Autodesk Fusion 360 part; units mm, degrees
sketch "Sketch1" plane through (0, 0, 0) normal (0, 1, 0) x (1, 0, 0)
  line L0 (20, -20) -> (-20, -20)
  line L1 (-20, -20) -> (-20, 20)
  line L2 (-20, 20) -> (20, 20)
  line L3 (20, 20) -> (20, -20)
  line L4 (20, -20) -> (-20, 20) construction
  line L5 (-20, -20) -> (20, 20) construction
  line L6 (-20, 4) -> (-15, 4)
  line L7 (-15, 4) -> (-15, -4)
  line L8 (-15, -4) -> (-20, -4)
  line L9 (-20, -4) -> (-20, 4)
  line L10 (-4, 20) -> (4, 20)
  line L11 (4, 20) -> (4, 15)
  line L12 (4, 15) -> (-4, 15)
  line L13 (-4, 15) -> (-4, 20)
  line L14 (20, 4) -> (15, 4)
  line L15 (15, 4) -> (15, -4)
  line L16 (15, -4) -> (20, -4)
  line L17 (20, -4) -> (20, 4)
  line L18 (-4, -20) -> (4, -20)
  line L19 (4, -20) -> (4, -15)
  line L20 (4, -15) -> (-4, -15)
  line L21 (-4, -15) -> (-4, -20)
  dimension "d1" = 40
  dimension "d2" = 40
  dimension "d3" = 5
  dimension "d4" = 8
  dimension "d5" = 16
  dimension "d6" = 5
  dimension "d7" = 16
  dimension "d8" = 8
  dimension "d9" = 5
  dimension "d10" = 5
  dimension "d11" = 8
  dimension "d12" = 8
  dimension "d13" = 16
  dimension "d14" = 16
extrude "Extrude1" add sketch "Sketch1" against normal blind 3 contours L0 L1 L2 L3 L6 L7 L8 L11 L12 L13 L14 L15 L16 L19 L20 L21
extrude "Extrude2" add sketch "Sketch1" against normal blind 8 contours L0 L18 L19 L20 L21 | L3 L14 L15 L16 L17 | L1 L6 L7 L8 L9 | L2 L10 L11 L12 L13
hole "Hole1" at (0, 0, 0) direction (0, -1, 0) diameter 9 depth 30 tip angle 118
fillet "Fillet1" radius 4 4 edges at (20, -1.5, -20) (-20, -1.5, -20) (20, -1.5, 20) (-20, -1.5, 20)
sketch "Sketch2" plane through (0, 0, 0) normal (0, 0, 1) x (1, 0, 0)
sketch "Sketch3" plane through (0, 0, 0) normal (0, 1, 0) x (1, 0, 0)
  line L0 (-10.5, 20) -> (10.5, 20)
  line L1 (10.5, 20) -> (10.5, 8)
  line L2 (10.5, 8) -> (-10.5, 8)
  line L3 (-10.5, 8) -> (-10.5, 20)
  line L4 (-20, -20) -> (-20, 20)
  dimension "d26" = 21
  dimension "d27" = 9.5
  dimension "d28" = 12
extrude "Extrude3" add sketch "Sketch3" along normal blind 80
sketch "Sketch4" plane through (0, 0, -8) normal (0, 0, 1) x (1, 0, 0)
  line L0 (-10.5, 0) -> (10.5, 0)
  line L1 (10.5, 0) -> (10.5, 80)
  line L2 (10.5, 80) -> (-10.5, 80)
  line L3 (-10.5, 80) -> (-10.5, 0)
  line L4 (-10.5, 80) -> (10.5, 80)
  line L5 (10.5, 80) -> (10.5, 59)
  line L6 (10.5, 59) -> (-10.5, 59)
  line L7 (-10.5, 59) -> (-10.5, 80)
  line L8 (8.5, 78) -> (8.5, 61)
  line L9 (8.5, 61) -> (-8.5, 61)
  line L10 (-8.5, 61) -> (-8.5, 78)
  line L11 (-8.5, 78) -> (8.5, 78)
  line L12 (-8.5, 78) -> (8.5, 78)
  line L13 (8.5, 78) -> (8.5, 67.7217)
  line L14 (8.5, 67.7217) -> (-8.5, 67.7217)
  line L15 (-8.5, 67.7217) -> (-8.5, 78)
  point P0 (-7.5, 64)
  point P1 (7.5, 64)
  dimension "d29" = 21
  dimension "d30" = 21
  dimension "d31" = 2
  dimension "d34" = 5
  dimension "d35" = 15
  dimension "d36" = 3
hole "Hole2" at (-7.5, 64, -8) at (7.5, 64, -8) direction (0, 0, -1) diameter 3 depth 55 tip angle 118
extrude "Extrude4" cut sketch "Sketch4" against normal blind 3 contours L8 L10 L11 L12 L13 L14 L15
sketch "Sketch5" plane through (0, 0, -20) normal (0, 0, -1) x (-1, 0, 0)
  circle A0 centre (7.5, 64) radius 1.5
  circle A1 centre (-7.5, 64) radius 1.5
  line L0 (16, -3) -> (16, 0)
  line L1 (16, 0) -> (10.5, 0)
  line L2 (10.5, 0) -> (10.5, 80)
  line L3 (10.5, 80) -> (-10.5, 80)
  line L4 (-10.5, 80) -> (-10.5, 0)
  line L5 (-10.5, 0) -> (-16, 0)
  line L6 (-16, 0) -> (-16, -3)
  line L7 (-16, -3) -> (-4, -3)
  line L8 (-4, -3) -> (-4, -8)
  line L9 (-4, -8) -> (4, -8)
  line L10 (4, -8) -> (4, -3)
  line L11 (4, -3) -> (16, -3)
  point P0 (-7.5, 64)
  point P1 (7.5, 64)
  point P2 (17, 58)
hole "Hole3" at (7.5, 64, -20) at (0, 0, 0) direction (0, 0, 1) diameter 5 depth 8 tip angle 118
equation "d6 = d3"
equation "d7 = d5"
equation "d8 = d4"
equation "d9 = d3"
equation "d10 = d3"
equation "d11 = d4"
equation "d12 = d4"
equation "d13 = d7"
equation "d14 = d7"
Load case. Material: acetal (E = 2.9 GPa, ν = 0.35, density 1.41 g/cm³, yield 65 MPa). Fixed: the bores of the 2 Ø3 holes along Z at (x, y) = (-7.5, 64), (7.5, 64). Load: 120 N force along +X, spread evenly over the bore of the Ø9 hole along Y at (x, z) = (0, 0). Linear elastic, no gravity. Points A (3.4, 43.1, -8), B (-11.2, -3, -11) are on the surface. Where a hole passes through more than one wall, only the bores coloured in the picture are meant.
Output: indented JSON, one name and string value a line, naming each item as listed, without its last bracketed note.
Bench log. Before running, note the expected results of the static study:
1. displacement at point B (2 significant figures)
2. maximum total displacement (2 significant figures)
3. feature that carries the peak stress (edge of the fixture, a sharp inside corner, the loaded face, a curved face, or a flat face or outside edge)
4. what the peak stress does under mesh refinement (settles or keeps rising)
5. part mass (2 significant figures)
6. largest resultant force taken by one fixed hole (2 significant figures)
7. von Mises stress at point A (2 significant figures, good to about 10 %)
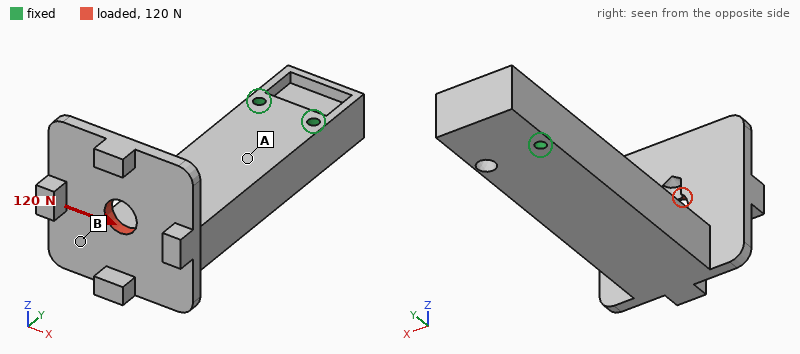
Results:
{
  "displacement at point B": "0.64 mm",
  "maximum total displacement": "1.2 mm",
  "feature that carries the peak stress": "edge of the fixture",
  "what the peak stress does under mesh refinement": "keeps rising",
  "part mass": "35 g",
  "largest resultant force taken by one fixed hole": "460 N",
  "von Mises stress at point A": "5.4 MPa"
}
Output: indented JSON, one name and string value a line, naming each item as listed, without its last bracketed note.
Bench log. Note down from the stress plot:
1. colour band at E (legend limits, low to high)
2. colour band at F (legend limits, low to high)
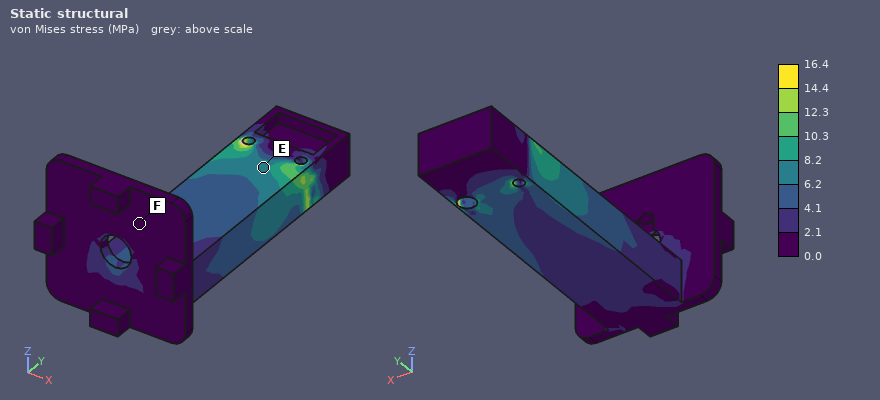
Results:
{
  "colour band at E": "6.2 to 8.2 MPa",
  "colour band at F": "0.0 to 2.1 MPa"
}
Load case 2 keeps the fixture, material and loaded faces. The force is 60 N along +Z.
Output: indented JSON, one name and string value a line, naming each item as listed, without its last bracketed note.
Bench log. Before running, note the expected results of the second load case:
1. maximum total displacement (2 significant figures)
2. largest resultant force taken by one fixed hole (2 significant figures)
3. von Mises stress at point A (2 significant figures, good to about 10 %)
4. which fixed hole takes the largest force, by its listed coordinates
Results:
{
  "maximum total displacement": "1.1 mm",
  "largest resultant force taken by one fixed hole": "64 N",
  "von Mises stress at point A": "5.2 MPa",
  "which fixed hole takes the largest force, by its listed coordinates": "(-7.5, 64)"
}
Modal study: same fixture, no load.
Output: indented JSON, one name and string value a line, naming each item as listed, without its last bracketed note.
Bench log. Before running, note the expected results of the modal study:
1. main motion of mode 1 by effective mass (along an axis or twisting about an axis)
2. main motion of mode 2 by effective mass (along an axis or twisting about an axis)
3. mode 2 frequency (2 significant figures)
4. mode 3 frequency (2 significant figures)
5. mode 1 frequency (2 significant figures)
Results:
{
  "main motion of mode 1 by effective mass": "along Z",
  "main motion of mode 2 by effective mass": "along X",
  "mode 2 frequency": "580 Hz",
  "mode 3 frequency": "700 Hz",
  "mode 1 frequency": "350 Hz"
}
